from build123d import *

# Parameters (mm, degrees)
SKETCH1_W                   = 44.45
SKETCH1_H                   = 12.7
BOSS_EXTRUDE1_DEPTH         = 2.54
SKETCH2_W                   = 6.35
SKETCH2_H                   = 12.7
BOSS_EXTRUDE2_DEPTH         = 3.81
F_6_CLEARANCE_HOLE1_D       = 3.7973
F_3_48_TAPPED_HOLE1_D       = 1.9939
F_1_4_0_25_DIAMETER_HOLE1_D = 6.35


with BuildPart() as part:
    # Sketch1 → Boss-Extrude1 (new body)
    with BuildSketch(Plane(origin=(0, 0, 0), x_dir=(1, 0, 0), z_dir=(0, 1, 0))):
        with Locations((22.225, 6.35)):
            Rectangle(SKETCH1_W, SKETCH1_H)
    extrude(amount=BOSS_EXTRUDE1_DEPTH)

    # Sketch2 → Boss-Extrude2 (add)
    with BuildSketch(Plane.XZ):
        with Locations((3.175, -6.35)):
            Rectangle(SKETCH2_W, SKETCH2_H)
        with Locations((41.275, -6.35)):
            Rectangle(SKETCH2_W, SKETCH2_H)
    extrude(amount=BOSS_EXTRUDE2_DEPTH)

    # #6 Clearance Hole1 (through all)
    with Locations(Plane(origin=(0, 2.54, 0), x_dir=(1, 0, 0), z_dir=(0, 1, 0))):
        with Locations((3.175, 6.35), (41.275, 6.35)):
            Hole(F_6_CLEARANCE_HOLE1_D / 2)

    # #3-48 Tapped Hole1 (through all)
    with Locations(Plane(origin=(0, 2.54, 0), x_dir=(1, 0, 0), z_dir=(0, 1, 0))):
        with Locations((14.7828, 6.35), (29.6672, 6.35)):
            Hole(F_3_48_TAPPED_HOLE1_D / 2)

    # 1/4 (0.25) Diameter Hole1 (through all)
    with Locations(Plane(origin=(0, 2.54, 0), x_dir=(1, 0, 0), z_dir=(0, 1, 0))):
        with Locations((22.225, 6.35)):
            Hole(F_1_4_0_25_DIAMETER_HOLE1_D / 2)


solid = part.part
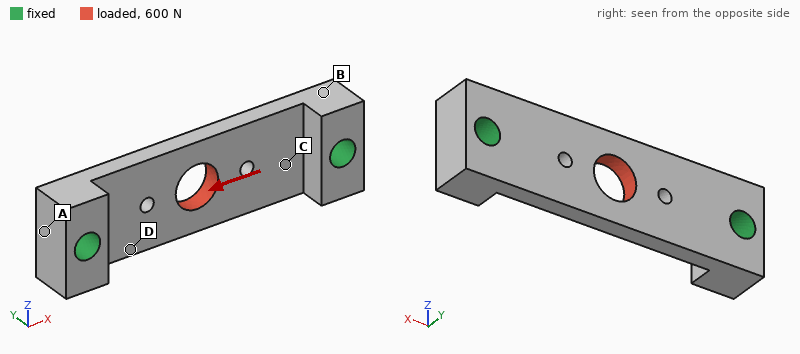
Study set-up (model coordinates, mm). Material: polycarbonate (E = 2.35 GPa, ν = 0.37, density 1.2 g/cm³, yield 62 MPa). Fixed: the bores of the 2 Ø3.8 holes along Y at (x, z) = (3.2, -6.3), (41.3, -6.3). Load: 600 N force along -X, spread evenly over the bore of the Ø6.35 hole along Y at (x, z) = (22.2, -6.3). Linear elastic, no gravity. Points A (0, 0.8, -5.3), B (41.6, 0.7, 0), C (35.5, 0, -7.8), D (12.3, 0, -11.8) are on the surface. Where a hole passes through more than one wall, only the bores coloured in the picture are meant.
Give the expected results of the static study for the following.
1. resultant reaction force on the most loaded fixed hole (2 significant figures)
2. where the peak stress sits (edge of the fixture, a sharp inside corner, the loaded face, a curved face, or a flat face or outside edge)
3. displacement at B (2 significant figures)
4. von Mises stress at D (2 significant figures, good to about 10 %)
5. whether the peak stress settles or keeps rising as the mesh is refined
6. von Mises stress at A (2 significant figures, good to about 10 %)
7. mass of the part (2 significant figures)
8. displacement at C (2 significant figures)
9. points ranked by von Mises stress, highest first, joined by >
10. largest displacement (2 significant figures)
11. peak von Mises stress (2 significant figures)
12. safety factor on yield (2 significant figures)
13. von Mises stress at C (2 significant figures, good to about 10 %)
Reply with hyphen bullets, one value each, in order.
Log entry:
- 300 N
- a curved face
- 17 µm
- 9.6 MPa
- settles
- 4.7 MPa
- 2.2 g
- 22 µm
- C > D > A > B
- 86 µm
- 35 MPa
- 1.8
- 13 MPa
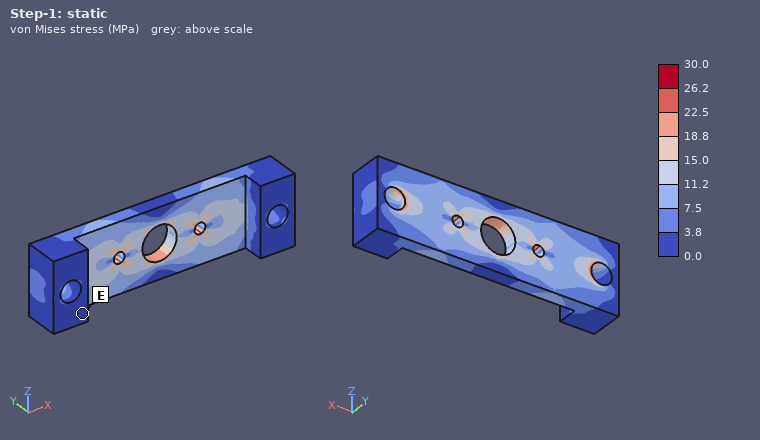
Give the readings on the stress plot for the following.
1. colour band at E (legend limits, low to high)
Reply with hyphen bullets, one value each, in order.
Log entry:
- 0.0 to 3.8 MPa
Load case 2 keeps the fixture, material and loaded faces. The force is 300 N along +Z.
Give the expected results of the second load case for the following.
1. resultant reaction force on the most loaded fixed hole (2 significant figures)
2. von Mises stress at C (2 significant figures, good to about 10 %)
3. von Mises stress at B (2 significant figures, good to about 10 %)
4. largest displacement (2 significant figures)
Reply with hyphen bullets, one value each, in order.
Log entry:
- 150 N
- 13 MPa
- 5.6 MPa
- 0.24 mm
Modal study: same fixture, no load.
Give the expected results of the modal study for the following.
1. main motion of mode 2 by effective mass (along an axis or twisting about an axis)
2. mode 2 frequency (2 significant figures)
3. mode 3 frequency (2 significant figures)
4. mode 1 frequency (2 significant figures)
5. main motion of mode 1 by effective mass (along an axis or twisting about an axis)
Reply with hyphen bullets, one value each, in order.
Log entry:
- twisting about X
- 5400 Hz
- 7800 Hz
- 3200 Hz
- along Y
